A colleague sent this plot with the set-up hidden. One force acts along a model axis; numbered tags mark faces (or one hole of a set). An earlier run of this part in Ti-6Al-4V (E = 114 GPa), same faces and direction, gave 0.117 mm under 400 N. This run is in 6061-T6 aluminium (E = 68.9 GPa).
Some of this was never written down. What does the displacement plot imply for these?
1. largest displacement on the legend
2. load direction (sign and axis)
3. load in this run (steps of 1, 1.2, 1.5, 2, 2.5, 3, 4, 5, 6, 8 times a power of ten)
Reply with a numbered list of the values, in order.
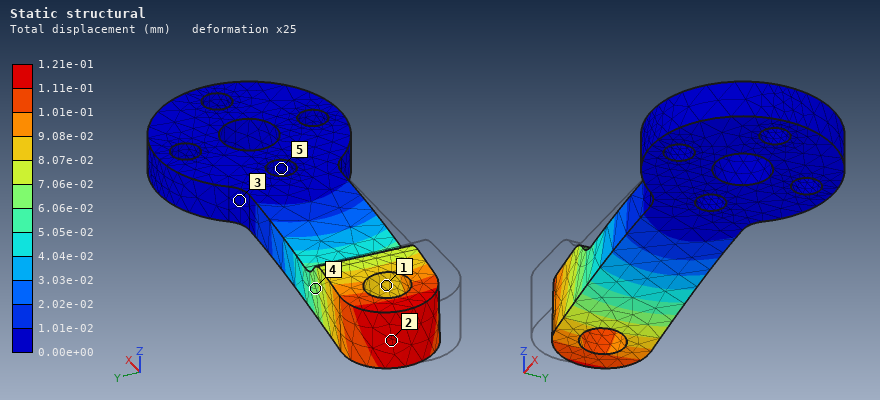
1. 1.21e-01 mm
2. +Y
3. 250 N
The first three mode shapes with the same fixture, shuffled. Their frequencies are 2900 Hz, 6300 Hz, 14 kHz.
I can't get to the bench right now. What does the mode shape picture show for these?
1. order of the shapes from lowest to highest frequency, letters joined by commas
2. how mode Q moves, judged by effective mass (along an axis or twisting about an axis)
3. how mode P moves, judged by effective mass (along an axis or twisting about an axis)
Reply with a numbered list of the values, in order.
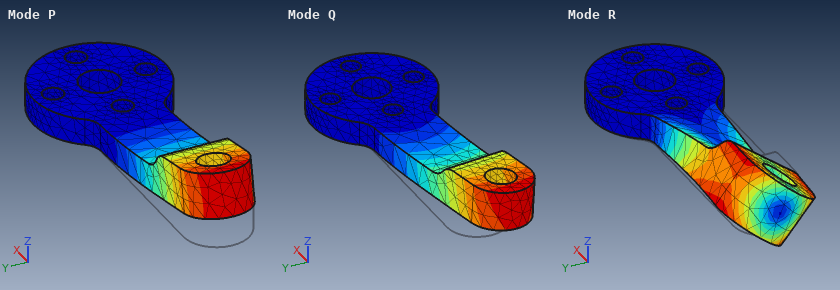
1. P, Q, R
2. along Y
3. along Z
